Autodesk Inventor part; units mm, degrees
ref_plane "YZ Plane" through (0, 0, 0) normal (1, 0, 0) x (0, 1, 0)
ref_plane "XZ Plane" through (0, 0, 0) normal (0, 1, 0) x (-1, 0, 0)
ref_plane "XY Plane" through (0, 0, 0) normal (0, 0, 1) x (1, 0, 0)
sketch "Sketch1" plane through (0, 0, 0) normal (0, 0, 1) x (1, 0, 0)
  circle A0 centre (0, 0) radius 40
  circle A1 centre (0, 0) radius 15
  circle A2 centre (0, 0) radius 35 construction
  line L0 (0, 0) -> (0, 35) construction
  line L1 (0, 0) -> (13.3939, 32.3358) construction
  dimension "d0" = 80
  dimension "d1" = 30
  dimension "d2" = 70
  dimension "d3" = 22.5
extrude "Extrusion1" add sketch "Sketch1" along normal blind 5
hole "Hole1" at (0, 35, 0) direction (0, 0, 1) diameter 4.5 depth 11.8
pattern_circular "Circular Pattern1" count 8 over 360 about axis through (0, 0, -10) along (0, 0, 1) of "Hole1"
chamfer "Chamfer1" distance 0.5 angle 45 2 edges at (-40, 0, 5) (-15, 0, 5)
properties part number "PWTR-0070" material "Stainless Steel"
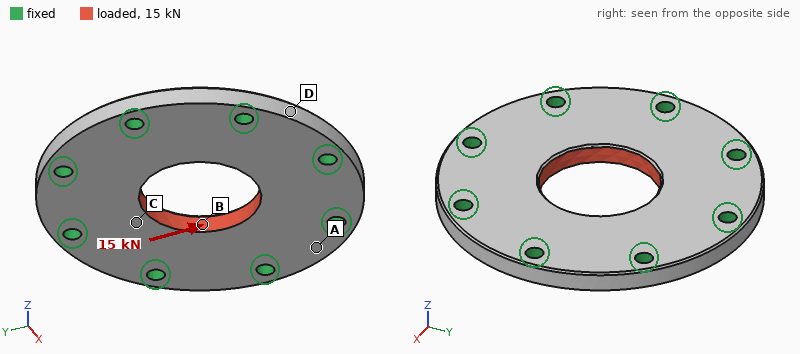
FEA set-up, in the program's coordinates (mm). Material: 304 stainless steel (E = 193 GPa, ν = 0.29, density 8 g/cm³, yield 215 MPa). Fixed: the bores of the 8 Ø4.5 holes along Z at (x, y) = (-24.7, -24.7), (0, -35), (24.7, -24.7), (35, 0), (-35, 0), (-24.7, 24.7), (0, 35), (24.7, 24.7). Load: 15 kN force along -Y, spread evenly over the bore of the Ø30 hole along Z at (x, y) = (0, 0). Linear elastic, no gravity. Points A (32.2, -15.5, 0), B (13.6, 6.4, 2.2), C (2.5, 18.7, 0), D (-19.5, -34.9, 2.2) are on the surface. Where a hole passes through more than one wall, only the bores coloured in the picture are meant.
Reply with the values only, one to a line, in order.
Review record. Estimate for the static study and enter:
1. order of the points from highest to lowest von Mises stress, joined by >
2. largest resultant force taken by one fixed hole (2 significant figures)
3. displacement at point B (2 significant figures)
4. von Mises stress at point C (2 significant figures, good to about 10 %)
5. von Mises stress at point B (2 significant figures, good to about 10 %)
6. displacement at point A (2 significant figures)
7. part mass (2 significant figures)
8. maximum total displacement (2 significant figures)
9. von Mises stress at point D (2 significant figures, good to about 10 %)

B > C > D > A
2.9 kN
4.1 µm
36 MPa
56 MPa
0.83 µm
170 g
4.2 µm
17 MPa
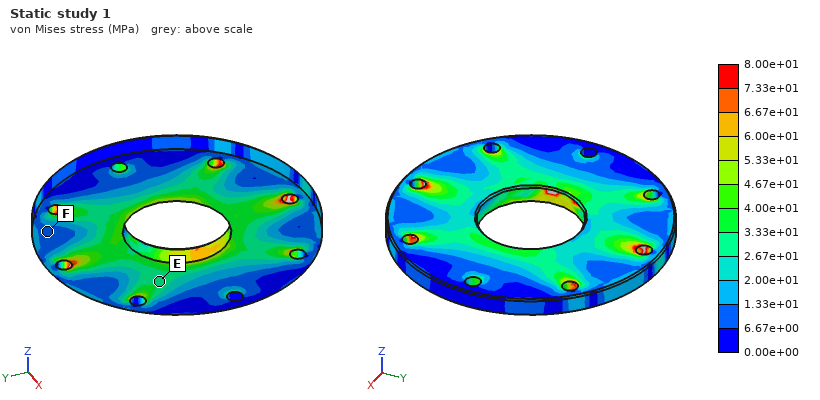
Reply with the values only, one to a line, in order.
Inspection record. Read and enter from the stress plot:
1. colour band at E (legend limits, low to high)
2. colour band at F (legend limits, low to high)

2.67e+01 to 3.33e+01 MPa
6.67e+00 to 1.33e+01 MPa
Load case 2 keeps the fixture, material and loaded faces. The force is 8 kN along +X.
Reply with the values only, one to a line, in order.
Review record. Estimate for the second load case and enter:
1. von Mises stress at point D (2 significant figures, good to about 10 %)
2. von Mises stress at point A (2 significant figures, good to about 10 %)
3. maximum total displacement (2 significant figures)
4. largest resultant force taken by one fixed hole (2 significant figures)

4.3 MPa
4.6 MPa
2.3 µm
1.5 kN
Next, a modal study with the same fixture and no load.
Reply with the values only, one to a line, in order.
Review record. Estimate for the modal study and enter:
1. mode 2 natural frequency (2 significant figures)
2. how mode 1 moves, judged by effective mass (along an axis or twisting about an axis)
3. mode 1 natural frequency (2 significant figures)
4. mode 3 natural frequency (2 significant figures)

16 kHz
along Z
12 kHz
16 kHz
